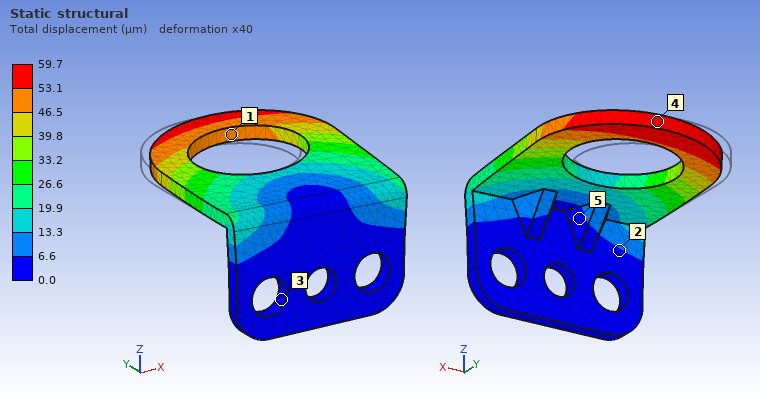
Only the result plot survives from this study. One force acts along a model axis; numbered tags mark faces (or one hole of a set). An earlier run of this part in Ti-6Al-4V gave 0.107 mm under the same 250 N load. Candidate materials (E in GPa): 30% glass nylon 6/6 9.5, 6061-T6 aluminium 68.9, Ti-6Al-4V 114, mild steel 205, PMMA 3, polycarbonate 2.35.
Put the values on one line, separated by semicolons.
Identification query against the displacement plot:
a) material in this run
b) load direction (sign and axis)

mild steel; +X
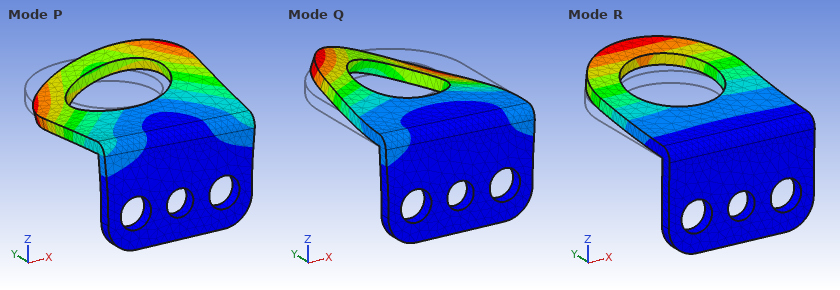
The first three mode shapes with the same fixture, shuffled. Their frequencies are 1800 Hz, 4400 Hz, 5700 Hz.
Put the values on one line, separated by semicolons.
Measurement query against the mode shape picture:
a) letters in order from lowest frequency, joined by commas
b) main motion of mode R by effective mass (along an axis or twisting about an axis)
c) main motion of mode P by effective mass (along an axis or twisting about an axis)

R, P, Q; along Z; along X
